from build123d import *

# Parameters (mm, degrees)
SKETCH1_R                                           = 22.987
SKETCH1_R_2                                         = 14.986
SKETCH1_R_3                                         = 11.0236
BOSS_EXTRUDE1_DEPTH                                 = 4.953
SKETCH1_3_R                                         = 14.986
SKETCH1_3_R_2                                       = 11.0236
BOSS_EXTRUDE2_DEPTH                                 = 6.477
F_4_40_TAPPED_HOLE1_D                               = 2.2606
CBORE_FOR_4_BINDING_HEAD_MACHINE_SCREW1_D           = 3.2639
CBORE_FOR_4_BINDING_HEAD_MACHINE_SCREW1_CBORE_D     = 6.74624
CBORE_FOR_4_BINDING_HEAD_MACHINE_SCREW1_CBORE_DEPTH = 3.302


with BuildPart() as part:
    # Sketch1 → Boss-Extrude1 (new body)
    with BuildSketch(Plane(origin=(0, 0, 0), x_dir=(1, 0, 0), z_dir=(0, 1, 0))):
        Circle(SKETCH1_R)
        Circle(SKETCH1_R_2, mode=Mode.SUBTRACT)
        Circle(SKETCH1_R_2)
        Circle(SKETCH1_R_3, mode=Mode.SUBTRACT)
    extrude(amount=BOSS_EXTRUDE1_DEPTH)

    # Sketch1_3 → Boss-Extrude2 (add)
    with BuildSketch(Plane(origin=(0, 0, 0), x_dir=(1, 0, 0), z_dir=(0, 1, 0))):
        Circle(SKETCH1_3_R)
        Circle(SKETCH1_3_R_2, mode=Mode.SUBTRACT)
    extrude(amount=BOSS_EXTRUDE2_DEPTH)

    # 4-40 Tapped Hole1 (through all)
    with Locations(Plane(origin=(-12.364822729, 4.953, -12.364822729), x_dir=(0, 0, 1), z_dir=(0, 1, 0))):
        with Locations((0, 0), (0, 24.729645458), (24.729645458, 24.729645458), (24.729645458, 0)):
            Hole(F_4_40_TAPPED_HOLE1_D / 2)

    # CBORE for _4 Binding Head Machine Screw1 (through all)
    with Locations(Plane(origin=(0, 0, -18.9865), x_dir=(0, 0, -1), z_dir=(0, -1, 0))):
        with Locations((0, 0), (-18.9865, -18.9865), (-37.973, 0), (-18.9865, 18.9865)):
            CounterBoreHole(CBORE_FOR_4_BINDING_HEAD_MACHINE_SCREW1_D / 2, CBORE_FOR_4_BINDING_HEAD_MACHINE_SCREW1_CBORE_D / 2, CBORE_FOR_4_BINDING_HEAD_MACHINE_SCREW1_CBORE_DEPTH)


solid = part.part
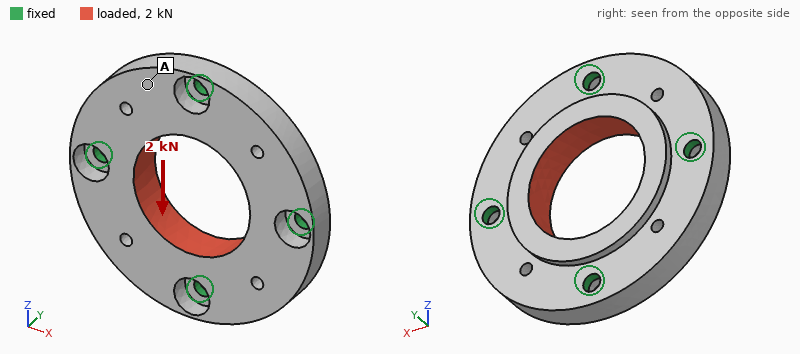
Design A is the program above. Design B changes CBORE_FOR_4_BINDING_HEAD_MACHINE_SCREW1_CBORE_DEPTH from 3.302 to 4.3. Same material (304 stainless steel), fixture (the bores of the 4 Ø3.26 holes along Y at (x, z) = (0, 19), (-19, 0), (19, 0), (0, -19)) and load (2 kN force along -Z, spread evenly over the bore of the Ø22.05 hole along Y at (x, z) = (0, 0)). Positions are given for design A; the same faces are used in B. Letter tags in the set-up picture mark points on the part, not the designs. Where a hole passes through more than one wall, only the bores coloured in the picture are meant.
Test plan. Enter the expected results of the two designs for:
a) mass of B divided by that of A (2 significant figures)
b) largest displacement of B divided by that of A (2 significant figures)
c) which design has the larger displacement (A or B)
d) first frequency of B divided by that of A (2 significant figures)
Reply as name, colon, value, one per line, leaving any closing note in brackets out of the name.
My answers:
mass of B divided by that of A: 0.98
largest displacement of B divided by that of A: 2.0
which design has the larger displacement: B
first frequency of B divided by that of A: 0.81
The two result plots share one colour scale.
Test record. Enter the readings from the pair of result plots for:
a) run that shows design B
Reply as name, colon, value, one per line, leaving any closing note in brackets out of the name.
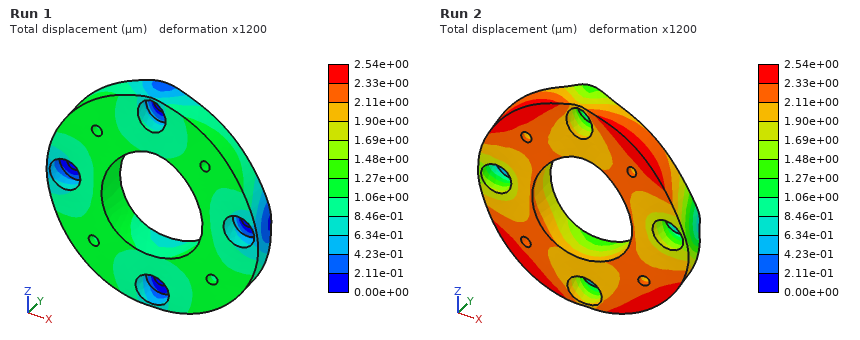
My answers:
run that shows design B: Run 2
